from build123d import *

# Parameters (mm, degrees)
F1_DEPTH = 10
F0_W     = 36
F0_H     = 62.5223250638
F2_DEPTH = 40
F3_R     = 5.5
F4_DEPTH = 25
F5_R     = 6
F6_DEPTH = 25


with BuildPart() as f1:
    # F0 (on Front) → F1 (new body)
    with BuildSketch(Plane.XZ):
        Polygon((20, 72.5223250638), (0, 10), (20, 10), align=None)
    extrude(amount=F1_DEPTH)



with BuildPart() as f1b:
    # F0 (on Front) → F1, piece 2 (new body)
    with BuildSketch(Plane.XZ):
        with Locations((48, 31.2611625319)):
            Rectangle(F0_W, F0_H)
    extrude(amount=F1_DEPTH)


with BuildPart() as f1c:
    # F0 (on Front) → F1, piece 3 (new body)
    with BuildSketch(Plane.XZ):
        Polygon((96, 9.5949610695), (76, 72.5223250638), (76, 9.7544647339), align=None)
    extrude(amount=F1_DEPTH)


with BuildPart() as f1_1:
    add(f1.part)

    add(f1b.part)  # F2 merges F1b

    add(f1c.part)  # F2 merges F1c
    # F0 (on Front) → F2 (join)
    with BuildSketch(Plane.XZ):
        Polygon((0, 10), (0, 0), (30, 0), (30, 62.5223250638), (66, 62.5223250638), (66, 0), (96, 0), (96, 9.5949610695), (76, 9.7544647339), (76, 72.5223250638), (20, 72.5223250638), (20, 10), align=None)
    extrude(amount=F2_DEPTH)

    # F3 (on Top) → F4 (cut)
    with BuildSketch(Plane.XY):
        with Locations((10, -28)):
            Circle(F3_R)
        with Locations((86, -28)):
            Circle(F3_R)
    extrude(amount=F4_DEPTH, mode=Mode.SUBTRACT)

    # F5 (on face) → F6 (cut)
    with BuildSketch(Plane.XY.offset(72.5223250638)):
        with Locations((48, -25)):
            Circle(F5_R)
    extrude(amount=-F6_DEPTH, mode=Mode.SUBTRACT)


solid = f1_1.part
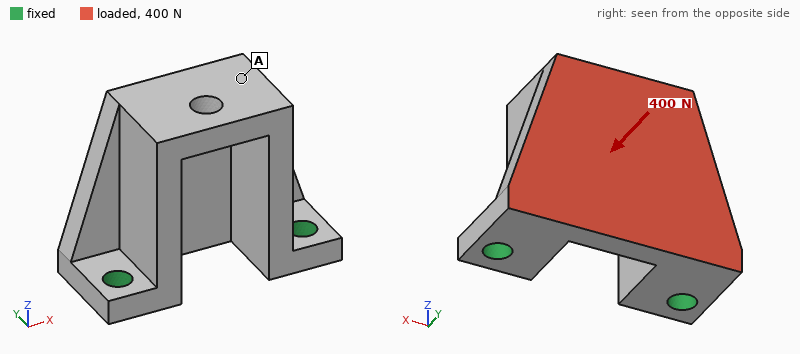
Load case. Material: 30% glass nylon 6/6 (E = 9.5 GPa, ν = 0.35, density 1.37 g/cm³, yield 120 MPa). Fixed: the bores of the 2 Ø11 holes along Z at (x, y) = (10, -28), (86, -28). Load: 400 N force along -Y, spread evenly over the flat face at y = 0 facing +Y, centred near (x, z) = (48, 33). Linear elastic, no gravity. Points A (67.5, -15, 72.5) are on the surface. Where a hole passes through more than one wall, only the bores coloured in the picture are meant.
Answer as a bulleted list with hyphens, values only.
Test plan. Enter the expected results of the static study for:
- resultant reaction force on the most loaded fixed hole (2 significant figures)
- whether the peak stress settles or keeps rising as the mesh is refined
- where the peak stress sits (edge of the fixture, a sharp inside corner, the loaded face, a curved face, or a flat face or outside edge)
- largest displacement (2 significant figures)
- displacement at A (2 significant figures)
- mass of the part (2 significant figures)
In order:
- 210 N
- keeps rising
- edge of the fixture
- 0.10 mm
- 0.099 mm
- 160 g
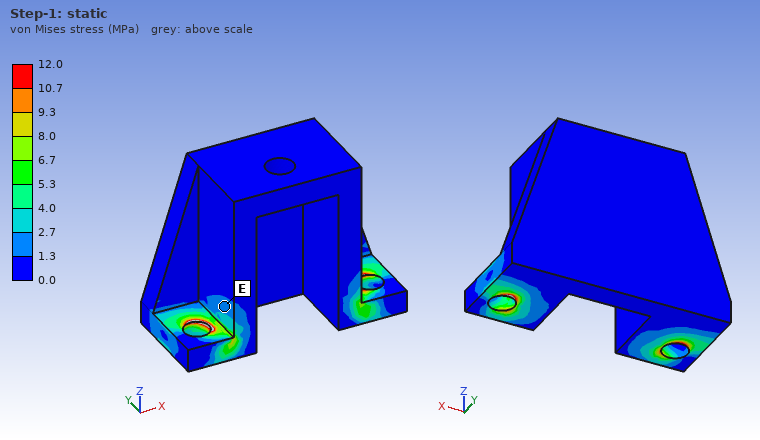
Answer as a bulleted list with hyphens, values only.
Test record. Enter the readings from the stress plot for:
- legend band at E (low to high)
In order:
- 1.3 to 2.7 MPa
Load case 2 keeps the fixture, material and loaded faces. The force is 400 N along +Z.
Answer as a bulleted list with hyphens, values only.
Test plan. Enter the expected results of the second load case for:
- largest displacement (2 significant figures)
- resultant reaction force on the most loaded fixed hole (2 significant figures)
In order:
- 89 µm
- 200 N
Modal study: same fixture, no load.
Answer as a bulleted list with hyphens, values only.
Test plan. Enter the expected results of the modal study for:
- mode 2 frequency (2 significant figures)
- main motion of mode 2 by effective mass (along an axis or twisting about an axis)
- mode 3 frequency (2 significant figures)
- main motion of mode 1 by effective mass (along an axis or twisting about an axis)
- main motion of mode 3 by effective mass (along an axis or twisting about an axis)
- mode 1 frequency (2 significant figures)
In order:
- 1400 Hz
- along X
- 3100 Hz
- along Y
- along X
- 860 Hz
